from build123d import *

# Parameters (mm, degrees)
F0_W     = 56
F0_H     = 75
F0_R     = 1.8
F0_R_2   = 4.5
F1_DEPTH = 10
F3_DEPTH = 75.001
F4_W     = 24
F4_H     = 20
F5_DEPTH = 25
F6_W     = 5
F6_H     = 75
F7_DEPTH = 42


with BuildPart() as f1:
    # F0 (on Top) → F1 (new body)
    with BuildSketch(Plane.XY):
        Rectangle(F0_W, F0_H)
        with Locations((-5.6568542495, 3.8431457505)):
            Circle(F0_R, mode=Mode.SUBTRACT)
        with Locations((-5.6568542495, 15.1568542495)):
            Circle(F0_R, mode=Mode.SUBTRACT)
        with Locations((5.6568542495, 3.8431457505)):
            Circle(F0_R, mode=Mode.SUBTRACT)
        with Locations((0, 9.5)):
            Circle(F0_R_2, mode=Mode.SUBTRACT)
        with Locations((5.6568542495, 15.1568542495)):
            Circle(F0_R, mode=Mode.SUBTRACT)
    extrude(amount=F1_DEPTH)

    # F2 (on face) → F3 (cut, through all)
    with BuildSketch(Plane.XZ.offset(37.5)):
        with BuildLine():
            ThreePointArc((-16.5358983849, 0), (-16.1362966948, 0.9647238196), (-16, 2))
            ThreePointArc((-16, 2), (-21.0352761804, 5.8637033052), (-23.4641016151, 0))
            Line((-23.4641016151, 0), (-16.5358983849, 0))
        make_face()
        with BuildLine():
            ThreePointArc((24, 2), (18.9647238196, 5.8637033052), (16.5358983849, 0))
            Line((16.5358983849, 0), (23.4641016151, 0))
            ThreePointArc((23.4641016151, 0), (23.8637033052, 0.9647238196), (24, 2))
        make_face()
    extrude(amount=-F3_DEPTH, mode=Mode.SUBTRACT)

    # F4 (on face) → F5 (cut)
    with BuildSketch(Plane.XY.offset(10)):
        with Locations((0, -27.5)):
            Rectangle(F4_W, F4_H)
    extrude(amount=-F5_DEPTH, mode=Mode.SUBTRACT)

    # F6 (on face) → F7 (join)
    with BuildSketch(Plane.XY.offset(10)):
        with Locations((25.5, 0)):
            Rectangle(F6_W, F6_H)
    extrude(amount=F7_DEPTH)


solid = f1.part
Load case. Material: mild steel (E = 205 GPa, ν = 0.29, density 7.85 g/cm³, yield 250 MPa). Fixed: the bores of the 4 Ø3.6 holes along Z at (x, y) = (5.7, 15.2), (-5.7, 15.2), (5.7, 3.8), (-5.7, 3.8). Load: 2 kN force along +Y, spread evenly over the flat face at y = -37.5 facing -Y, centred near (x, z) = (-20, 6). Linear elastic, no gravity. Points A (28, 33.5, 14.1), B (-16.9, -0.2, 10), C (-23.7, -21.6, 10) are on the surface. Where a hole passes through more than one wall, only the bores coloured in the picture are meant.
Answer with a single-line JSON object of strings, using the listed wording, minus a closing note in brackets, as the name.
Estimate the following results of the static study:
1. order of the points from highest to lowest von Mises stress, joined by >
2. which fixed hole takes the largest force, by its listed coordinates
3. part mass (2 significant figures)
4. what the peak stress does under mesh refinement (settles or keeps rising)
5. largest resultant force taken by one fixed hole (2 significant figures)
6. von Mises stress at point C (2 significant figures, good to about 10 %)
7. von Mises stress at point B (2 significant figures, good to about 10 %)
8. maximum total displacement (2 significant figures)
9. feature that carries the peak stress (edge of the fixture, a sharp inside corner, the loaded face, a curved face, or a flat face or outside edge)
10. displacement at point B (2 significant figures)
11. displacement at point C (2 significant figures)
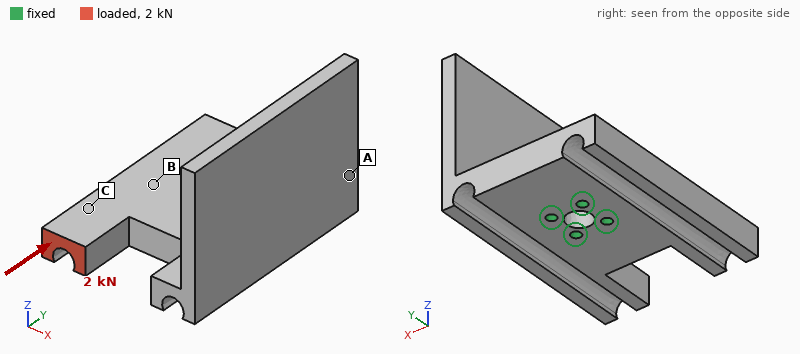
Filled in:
{"order of the points from highest to lowest von Mises stress, joined by >": "C > B > A", "which fixed hole takes the largest force, by its listed coordinates": "(-5.7, 3.8)", "part mass": "360 g", "what the peak stress does under mesh refinement": "keeps rising", "largest resultant force taken by one fixed hole": "1.8 kN", "von Mises stress at point C": "17 MPa", "von Mises stress at point B": "13 MPa", "maximum total displacement": "8.9 µm", "feature that carries the peak stress": "edge of the fixture", "displacement at point B": "1.7 µm", "displacement at point C": "5.5 µm"}
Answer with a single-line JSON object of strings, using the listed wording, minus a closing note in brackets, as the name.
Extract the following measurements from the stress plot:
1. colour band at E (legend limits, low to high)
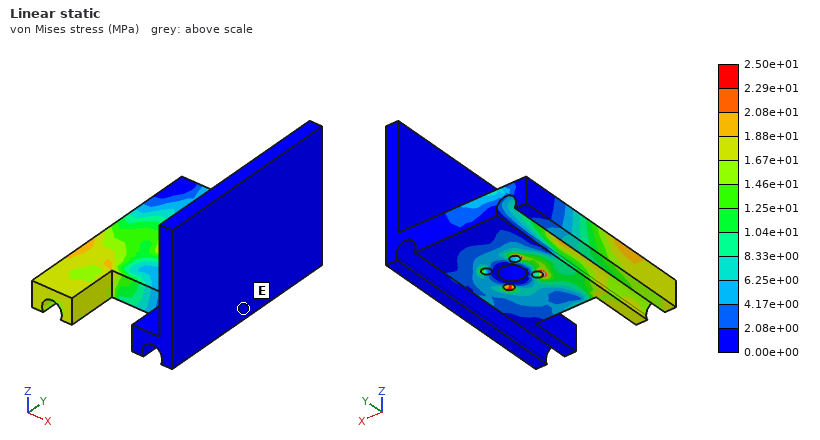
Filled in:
{"colour band at E": "0.00e+00 to 2.08e+00 MPa"}
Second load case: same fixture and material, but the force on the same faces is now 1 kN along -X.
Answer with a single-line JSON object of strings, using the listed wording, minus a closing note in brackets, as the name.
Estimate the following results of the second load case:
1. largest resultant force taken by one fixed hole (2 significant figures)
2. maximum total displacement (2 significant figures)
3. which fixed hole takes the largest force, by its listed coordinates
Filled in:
{"largest resultant force taken by one fixed hole": "1.7 kN", "maximum total displacement": "31 µm", "which fixed hole takes the largest force, by its listed coordinates": "(5.7, 3.8)"}
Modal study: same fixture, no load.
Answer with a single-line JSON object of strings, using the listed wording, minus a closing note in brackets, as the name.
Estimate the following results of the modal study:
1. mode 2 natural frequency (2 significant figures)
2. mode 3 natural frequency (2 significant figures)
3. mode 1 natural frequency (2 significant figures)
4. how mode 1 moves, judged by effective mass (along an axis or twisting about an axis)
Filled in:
{"mode 2 natural frequency": "2400 Hz", "mode 3 natural frequency": "3200 Hz", "mode 1 natural frequency": "1300 Hz", "how mode 1 moves, judged by effective mass": "along X"}
